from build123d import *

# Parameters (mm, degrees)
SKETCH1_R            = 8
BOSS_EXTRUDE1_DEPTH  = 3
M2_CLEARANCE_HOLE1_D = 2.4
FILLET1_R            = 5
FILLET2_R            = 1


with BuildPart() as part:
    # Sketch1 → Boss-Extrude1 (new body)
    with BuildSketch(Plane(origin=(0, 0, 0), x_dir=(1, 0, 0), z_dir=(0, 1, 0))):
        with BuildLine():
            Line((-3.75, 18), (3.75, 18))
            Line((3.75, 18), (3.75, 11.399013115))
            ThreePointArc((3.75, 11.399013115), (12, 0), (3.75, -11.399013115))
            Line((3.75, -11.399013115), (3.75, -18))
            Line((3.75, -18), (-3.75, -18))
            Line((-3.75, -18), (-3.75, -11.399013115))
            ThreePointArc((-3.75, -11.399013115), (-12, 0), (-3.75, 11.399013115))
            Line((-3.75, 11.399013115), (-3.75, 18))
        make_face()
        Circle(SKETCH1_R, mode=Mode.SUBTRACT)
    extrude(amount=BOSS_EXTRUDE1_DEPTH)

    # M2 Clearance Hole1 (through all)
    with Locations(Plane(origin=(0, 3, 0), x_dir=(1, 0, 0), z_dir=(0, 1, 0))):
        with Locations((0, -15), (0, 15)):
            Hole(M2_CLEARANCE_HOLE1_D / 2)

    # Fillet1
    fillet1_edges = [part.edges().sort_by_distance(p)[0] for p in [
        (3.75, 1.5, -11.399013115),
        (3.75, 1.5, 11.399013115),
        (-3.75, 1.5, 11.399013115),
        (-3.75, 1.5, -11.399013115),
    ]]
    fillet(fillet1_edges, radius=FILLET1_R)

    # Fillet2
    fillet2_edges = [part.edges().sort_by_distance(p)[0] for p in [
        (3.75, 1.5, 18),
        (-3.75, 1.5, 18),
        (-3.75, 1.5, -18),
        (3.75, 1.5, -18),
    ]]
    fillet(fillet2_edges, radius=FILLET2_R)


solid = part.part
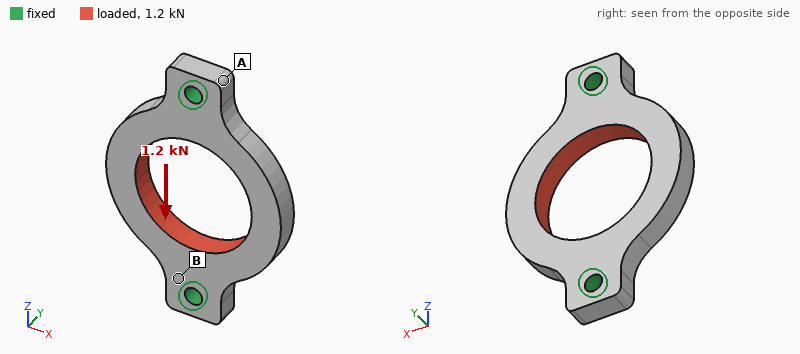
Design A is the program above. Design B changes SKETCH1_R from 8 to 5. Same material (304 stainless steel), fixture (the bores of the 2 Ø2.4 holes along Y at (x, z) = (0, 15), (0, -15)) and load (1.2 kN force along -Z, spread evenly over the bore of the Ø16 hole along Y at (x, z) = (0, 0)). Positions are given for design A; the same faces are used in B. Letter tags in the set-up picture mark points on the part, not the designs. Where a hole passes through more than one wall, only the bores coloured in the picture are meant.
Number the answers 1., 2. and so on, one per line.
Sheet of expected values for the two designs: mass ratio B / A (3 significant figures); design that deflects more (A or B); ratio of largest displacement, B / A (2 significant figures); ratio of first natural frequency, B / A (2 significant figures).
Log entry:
1. 1.36
2. A
3. 0.53
4. 0.97
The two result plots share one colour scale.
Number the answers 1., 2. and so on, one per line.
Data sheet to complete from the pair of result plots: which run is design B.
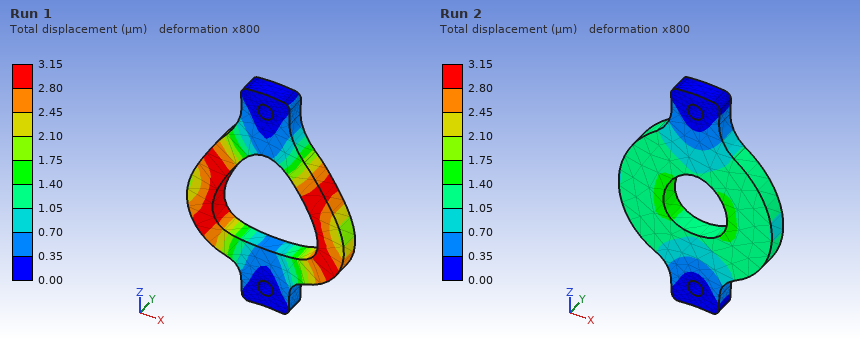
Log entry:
1. Run 2
